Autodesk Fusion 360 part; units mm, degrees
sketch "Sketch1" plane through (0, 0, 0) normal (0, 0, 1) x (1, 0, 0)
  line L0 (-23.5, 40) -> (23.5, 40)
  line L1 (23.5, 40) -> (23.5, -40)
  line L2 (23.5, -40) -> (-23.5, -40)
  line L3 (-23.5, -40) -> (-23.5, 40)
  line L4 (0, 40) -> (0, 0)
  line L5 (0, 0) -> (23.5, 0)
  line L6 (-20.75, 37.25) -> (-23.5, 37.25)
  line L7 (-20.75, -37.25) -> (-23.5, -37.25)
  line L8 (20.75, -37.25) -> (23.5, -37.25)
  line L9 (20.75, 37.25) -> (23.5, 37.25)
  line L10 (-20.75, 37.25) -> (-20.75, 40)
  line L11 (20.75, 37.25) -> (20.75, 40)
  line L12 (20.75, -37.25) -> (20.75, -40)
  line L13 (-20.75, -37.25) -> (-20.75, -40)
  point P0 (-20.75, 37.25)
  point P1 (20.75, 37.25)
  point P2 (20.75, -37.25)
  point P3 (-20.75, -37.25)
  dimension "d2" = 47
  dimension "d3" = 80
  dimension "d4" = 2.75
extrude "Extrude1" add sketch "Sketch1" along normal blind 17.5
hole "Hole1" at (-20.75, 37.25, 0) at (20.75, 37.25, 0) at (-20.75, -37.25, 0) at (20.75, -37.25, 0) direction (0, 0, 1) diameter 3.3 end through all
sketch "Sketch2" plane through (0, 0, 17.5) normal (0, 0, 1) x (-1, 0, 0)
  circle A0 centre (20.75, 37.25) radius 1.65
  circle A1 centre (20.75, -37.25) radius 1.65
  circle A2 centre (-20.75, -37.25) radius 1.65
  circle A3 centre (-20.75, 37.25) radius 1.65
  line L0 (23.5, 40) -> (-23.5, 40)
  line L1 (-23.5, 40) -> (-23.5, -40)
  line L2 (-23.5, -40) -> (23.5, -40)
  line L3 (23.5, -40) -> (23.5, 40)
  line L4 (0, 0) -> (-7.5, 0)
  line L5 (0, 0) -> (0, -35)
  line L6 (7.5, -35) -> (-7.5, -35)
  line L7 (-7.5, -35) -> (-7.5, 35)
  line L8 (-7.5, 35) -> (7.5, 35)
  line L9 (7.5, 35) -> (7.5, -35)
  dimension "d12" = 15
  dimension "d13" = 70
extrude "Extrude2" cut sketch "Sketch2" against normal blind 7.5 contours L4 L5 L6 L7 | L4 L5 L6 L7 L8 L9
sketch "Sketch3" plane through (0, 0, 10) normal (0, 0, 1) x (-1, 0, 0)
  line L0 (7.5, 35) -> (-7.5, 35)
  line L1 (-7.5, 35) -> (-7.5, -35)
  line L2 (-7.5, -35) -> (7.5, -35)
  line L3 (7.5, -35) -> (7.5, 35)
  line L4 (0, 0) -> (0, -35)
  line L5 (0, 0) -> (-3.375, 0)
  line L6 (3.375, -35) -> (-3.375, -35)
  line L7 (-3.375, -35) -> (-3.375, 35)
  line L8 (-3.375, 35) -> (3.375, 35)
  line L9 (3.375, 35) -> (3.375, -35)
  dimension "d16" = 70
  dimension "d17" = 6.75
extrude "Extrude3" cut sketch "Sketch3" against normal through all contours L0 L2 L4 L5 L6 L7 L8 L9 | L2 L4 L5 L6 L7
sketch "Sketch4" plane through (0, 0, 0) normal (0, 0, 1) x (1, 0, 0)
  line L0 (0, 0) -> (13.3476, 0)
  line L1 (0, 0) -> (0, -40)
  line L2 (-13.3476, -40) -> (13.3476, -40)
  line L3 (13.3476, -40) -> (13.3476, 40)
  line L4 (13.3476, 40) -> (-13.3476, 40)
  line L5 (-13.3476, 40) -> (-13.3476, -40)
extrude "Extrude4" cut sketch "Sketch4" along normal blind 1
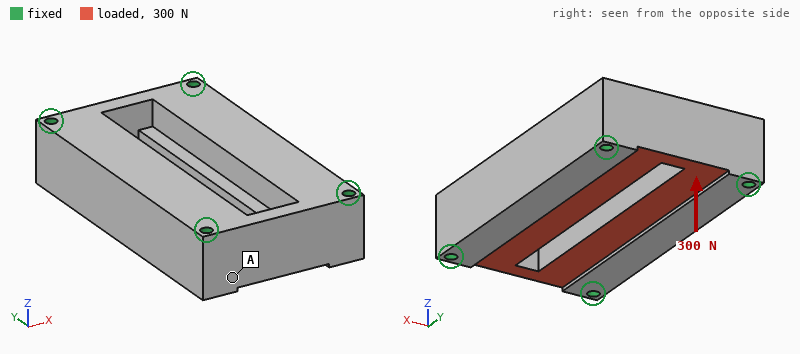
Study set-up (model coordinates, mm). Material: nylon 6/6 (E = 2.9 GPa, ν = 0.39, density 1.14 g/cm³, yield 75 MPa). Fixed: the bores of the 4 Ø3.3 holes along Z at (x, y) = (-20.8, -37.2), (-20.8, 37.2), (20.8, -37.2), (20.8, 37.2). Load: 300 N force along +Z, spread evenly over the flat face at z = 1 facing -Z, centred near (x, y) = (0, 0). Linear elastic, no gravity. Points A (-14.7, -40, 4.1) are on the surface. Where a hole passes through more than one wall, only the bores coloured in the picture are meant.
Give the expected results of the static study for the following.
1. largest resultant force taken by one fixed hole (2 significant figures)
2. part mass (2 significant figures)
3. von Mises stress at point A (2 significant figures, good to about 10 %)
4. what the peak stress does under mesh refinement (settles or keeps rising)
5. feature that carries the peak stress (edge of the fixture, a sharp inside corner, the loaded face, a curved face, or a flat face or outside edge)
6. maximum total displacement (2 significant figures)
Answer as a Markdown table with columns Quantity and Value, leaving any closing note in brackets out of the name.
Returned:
| Quantity | Value |
|---|---|
| largest resultant force taken by one fixed hole | 75 N |
| part mass | 58 g |
| von Mises stress at point A | 0.44 MPa |
| what the peak stress does under mesh refinement | keeps rising |
| feature that carries the peak stress | edge of the fixture |
| maximum total displacement | 30 µm |
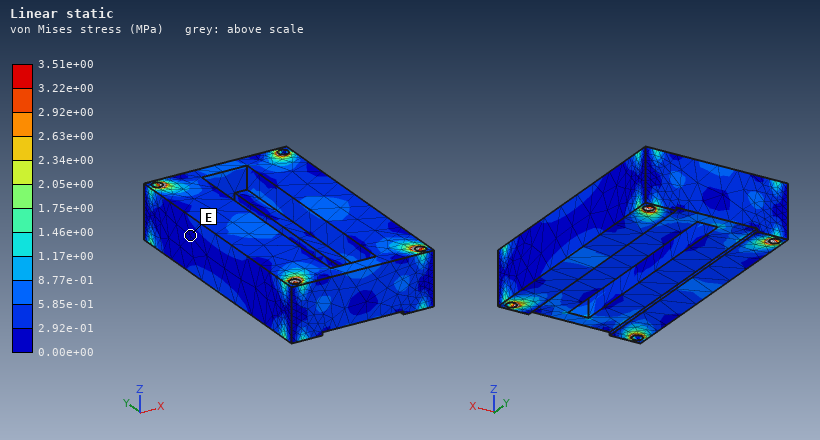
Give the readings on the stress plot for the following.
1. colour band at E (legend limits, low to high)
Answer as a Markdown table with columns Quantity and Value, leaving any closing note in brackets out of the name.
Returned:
| Quantity | Value |
|---|---|
| colour band at E | 0.00e+00 to 2.92e-01 MPa |
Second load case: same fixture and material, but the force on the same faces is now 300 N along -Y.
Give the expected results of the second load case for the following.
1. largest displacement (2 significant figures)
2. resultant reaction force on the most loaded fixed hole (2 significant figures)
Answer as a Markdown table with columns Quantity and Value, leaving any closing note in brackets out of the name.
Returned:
| Quantity | Value |
|---|---|
| largest displacement | 8.0 µm |
| resultant reaction force on the most loaded fixed hole | 79 N |
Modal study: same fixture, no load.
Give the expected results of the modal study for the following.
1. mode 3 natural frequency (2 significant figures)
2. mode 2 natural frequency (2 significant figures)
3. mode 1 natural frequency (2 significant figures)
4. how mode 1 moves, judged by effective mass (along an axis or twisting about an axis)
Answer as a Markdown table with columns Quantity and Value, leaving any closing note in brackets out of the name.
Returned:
| Quantity | Value |
|---|---|
| mode 3 natural frequency | 3200 Hz |
| mode 2 natural frequency | 3200 Hz |
| mode 1 natural frequency | 3100 Hz |
| how mode 1 moves, judged by effective mass | along Z |
